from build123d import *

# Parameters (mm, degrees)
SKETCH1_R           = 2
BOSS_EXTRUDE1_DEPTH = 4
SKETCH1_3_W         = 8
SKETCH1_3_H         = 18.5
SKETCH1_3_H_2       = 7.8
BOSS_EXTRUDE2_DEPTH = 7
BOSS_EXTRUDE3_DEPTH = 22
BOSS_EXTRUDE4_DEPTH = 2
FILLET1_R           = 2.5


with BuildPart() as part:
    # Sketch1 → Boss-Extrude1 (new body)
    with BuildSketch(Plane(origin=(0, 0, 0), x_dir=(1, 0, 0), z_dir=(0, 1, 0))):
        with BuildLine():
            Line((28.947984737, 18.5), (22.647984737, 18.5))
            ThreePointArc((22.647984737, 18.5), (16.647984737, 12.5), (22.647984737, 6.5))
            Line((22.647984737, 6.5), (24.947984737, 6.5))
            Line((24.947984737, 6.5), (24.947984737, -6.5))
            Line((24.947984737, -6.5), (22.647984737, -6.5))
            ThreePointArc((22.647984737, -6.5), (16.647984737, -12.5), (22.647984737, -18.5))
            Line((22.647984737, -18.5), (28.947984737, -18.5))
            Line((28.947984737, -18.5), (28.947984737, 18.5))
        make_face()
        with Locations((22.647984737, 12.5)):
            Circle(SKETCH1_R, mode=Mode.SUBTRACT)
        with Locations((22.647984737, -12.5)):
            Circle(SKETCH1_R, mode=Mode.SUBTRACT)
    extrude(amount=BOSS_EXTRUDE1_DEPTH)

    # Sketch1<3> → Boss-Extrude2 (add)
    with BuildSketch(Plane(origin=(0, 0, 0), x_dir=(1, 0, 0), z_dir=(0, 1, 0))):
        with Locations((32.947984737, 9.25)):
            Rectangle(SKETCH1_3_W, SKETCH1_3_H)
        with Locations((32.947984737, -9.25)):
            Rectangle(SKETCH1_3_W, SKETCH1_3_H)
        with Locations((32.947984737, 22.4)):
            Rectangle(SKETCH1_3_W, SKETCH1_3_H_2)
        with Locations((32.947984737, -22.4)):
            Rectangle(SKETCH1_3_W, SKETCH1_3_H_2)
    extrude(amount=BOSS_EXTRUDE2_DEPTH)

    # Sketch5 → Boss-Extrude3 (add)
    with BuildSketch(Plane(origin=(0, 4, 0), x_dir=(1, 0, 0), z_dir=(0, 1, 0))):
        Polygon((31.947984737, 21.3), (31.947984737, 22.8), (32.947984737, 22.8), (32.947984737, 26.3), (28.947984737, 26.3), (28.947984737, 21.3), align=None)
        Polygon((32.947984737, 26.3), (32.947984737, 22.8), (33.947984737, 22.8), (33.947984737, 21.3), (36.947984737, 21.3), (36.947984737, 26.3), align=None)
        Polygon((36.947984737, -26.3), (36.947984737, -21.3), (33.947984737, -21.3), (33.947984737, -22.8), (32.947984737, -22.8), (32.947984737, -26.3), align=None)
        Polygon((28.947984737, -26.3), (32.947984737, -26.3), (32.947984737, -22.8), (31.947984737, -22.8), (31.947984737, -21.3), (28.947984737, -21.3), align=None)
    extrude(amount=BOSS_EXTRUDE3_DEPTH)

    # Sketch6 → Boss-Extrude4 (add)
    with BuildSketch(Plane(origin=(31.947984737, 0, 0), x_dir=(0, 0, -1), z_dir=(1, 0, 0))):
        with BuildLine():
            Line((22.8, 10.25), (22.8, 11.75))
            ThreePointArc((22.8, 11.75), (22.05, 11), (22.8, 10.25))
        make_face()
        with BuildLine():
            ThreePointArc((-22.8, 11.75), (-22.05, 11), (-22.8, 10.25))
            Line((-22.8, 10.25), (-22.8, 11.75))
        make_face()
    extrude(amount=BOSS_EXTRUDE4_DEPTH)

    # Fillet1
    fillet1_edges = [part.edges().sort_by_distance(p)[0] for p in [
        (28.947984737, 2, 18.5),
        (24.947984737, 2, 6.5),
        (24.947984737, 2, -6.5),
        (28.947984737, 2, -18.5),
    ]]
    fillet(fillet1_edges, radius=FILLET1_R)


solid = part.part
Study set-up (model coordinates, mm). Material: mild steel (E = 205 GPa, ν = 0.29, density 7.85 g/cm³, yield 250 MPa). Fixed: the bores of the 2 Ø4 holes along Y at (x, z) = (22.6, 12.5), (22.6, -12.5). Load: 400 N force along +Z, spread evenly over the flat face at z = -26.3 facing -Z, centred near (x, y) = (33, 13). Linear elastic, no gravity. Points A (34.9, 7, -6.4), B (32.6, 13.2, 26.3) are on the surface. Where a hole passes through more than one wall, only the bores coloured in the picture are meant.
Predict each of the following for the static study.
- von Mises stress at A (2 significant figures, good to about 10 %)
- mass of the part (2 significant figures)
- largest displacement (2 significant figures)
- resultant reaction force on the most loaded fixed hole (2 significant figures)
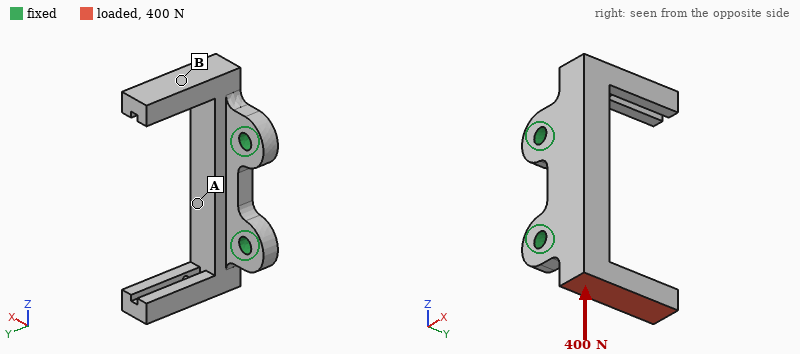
31 MPa
43 g
58 µm
290 N
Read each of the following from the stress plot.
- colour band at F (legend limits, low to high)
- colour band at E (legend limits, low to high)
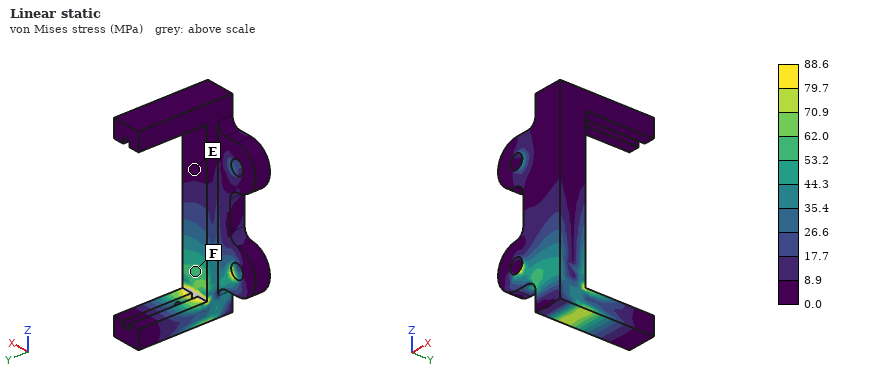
53.2 to 62.0 MPa
0.0 to 8.9 MPa
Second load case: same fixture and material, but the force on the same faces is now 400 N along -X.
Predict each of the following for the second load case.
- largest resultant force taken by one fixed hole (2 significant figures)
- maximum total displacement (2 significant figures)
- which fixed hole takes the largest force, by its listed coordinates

610 N
77 µm
(22.6, -12.5)
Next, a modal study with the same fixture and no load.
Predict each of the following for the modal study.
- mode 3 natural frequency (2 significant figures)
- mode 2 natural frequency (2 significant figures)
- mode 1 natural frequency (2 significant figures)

5600 Hz
4800 Hz
4300 Hz
